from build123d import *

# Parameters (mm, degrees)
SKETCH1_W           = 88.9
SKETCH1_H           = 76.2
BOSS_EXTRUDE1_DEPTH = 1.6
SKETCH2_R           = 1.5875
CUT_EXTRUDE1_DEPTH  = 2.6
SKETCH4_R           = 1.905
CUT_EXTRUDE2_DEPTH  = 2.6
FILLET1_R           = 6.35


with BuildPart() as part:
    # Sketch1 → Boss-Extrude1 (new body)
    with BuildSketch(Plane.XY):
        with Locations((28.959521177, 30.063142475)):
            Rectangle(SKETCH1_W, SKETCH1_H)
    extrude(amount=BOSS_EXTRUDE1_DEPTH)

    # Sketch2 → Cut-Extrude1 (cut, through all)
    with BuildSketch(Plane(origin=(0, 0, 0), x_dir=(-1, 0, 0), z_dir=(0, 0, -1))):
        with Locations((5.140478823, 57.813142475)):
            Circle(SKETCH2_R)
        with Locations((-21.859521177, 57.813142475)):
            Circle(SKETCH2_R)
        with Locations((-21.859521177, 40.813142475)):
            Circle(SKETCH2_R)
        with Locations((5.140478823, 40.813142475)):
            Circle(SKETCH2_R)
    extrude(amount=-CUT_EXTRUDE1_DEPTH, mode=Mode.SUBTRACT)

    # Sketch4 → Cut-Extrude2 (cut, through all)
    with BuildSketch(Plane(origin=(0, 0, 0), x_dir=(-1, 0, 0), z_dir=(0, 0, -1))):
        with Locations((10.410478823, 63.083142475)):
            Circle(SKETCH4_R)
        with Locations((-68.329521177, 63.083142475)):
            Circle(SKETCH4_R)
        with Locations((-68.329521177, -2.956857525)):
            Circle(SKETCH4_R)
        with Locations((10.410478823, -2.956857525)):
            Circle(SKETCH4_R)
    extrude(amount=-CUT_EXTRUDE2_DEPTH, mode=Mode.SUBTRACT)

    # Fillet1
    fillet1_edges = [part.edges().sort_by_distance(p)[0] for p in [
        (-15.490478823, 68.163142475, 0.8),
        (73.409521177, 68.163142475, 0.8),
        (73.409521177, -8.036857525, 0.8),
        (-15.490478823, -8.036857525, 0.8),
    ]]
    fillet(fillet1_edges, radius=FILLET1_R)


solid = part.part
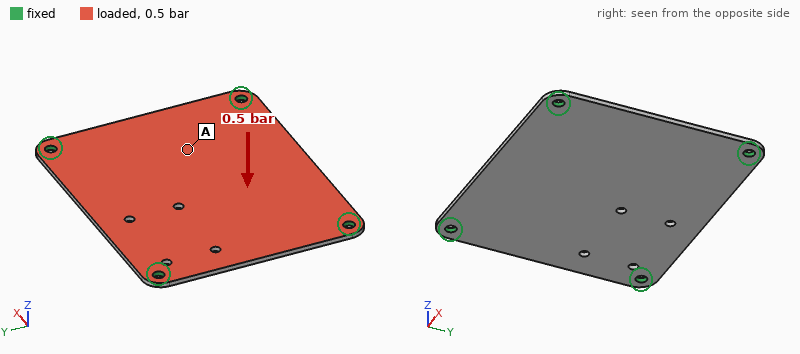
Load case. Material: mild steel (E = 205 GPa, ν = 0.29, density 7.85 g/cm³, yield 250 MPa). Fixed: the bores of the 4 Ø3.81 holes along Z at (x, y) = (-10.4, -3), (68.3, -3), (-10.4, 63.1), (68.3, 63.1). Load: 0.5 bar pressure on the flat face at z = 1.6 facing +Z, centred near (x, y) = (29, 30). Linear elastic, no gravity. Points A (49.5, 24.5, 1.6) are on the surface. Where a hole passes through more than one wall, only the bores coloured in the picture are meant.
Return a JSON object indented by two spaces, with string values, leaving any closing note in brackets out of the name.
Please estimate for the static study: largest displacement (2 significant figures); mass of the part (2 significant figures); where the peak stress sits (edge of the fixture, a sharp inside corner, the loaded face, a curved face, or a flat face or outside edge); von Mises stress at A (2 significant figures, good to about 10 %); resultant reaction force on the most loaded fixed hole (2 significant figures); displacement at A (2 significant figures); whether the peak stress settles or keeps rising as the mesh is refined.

{
  "largest displacement": "0.14 mm",
  "mass of the part": "84 g",
  "where the peak stress sits": "edge of the fixture",
  "von Mises stress at A": "26 MPa",
  "resultant reaction force on the most loaded fixed hole": "84 N",
  "displacement at A": "0.11 mm",
  "whether the peak stress settles or keeps rising as the mesh is refined": "keeps rising"
}
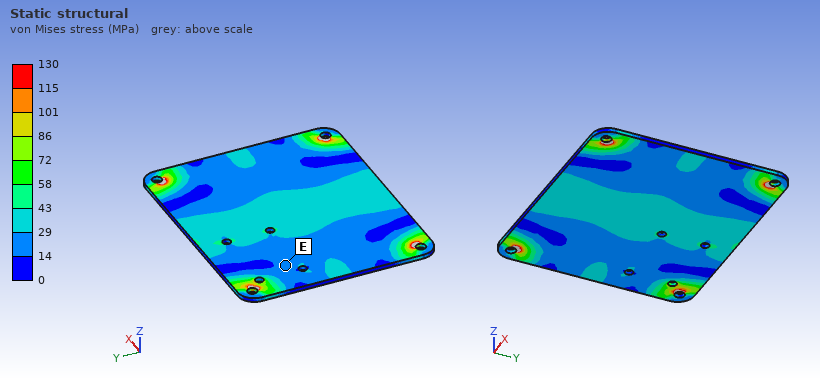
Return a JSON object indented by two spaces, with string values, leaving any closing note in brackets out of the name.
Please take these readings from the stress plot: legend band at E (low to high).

{
  "legend band at E": "14 to 29 MPa"
}
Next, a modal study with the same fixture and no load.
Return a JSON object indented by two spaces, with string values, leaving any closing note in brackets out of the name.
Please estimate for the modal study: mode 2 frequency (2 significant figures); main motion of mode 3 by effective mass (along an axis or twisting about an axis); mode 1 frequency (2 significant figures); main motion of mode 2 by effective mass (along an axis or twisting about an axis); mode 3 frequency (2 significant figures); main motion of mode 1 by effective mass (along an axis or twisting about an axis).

{
  "mode 2 frequency": "1600 Hz",
  "main motion of mode 3 by effective mass": "twisting about Y",
  "mode 1 frequency": "1000 Hz",
  "main motion of mode 2 by effective mass": "twisting about X",
  "mode 3 frequency": "2000 Hz",
  "main motion of mode 1 by effective mass": "along Z"
}
